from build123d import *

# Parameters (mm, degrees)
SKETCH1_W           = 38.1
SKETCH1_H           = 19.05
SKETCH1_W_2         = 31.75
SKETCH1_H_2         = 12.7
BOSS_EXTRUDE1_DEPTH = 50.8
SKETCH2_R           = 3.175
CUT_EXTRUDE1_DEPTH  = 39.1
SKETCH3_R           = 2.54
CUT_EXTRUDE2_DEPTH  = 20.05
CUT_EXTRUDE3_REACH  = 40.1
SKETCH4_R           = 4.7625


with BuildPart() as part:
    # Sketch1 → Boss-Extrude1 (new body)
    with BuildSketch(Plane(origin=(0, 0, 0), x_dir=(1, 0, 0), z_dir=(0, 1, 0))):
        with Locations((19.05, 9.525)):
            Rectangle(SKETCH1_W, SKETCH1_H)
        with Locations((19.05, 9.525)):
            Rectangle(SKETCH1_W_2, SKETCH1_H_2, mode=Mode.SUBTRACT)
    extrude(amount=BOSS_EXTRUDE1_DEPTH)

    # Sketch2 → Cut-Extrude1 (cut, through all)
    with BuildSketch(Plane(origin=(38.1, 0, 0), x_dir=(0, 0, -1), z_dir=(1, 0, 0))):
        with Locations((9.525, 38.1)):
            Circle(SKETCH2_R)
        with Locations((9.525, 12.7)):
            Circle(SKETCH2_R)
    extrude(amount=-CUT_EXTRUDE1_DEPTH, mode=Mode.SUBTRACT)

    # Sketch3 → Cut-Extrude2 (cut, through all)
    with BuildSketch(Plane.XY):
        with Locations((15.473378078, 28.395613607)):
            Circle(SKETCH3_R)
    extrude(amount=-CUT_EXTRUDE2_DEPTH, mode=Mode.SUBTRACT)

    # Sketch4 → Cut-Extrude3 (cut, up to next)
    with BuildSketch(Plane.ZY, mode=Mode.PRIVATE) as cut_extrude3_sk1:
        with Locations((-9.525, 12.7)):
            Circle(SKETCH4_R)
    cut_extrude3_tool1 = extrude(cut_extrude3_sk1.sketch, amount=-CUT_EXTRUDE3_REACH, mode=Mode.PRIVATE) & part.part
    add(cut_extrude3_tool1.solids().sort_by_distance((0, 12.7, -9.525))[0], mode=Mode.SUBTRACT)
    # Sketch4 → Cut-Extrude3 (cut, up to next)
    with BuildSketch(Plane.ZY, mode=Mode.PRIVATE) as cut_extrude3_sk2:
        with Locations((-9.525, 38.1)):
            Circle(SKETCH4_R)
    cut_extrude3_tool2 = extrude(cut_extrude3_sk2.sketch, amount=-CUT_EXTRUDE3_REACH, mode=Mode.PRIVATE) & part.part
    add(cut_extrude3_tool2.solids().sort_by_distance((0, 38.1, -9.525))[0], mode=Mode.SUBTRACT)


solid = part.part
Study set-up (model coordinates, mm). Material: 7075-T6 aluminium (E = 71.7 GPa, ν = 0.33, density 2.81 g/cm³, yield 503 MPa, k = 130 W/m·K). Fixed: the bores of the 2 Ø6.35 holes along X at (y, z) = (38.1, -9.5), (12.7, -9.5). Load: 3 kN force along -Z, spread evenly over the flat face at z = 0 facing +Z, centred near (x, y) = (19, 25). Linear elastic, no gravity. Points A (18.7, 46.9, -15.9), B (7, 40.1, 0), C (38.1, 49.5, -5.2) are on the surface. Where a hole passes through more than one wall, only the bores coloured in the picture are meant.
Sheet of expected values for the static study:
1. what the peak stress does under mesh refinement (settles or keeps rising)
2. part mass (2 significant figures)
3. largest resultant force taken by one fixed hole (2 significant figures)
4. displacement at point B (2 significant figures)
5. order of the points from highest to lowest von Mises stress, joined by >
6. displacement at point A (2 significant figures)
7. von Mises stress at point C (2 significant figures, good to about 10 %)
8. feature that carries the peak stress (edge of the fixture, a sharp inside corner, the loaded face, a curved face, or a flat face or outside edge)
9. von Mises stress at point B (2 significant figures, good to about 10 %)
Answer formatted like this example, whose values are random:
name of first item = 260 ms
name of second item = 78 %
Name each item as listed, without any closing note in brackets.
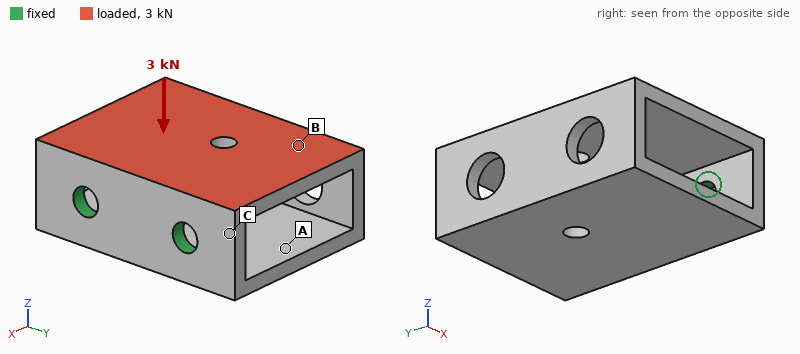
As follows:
what the peak stress does under mesh refinement = keeps rising
part mass = 44 g
largest resultant force taken by one fixed hole = 1.5 kN
displacement at point B = 0.60 mm
order of the points from highest to lowest von Mises stress, joined by > = C > B > A
displacement at point A = 0.32 mm
von Mises stress at point C = 160 MPa
feature that carries the peak stress = edge of the fixture
von Mises stress at point B = 88 MPa
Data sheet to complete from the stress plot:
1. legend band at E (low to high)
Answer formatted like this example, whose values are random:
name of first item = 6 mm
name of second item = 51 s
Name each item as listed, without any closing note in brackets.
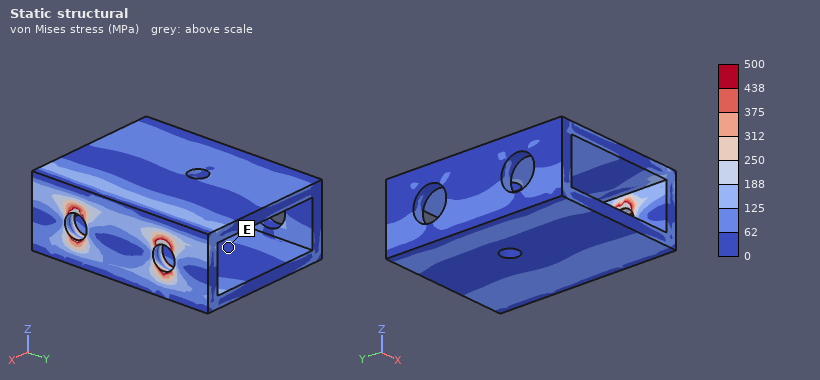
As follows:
legend band at E = 0 to 62 MPa
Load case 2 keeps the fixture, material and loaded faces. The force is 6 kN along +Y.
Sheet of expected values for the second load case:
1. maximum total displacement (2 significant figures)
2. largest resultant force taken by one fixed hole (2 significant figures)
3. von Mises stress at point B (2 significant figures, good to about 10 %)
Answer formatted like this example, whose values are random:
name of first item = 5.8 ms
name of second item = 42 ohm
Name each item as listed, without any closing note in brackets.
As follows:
maximum total displacement = 0.22 mm
largest resultant force taken by one fixed hole = 4.9 kN
von Mises stress at point B = 41 MPa
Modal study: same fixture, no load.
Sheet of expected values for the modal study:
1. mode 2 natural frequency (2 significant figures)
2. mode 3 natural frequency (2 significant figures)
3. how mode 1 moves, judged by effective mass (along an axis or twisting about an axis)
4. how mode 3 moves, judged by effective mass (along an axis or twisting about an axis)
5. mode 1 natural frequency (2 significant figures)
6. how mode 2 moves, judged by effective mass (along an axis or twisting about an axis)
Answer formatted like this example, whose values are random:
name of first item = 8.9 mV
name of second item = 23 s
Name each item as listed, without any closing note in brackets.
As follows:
mode 2 natural frequency = 5200 Hz
mode 3 natural frequency = 5700 Hz
how mode 1 moves, judged by effective mass = along Z
how mode 3 moves, judged by effective mass = along Y
mode 1 natural frequency = 1800 Hz
how mode 2 moves, judged by effective mass = twisting about X
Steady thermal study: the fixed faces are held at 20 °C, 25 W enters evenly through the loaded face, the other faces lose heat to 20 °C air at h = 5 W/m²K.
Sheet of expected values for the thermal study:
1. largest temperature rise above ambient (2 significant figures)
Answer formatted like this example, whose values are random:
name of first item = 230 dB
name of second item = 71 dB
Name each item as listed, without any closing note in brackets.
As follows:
largest temperature rise above ambient = 19 K
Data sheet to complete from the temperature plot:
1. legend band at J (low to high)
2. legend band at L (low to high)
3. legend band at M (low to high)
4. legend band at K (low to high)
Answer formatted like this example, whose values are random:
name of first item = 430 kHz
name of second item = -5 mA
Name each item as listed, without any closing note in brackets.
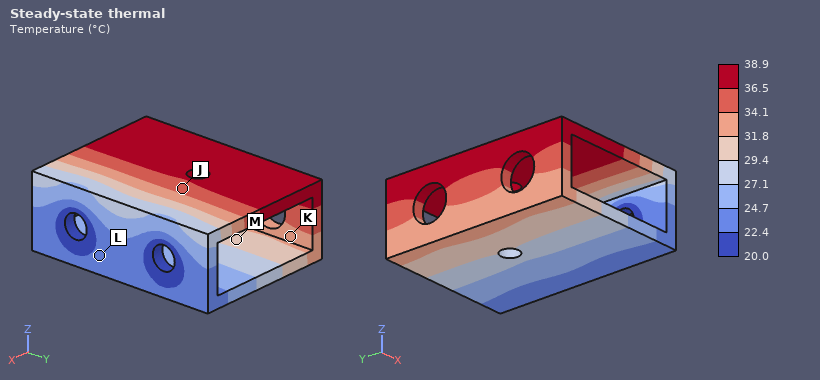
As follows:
legend band at J = 34.1 to 36.5 °C
legend band at L = 22.4 to 24.7 °C
legend band at M = 29.4 to 31.8 °C
legend band at K = 31.8 to 34.1 °C
